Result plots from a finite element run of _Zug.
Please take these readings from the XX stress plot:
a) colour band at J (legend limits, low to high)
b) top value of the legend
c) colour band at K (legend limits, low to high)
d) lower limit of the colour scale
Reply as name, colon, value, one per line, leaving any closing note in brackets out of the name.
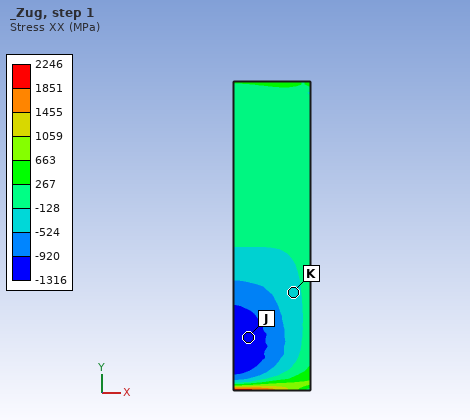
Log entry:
colour band at J: -1316 to -920 MPa
top value of the legend: 2246 MPa
colour band at K: -524 to -128 MPa
lower limit of the colour scale: -1316 MPa
